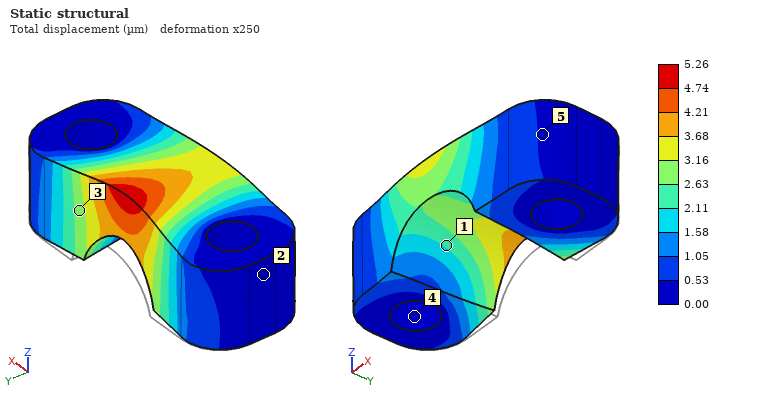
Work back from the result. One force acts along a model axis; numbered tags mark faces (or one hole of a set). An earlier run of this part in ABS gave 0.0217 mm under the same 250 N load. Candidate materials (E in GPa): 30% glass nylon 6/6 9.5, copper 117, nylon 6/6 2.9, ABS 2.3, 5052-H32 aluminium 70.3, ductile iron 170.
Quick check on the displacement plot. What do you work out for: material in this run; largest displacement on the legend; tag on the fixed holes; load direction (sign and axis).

30% glass nylon 6/6
5.26 µm
4
-Y
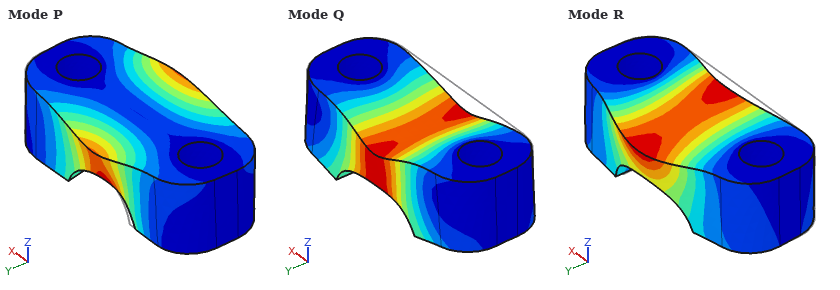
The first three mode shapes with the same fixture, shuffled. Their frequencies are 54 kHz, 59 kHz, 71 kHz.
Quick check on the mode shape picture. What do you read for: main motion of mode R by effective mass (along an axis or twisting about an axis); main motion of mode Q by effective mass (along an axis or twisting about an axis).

along Y
along Z
